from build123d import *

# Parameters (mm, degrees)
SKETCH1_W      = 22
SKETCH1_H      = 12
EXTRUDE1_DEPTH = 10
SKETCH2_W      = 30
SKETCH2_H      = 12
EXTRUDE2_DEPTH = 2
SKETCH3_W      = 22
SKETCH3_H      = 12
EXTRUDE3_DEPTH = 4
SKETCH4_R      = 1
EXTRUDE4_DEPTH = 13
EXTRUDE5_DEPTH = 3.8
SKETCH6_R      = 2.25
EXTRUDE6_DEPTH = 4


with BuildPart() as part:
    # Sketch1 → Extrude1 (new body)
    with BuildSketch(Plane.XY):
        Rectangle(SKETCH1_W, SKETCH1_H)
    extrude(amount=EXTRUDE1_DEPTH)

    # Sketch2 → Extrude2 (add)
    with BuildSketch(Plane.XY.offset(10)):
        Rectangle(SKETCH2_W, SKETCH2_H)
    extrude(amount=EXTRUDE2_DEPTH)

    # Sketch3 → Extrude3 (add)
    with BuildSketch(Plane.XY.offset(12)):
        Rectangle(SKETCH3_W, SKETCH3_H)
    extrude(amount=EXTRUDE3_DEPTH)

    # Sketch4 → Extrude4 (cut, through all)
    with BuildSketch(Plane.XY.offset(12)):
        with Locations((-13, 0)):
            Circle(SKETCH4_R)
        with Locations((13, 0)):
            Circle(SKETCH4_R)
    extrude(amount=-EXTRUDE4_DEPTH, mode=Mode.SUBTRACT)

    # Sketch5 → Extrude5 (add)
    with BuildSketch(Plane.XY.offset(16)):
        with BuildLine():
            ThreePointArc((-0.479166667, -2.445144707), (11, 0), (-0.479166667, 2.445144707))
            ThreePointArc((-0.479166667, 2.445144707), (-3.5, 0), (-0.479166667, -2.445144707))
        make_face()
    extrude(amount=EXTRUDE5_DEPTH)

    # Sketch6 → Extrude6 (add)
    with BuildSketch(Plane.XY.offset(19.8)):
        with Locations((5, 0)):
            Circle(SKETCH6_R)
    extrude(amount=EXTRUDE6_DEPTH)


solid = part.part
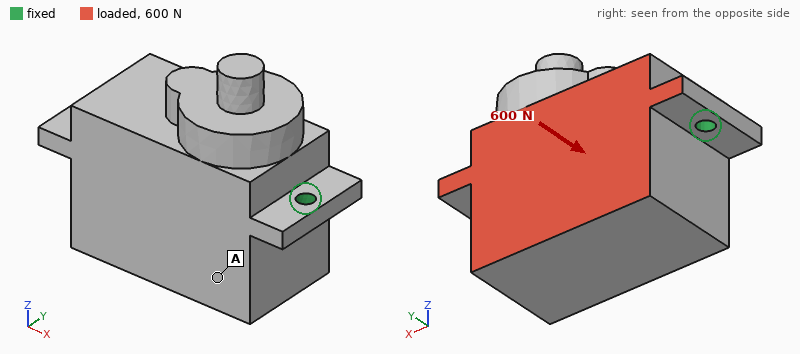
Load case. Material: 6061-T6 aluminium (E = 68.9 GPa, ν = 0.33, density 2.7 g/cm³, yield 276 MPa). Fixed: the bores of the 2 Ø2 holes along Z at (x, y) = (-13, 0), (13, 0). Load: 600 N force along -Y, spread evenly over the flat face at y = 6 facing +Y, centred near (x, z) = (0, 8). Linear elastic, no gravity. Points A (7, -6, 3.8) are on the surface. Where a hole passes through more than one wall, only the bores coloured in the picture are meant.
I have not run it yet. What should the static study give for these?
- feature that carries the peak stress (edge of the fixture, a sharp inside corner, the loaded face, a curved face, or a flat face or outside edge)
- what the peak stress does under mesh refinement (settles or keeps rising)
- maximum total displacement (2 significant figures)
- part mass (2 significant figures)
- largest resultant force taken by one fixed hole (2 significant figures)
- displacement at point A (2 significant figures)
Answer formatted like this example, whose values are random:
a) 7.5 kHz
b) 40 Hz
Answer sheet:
a) edge of the fixture
b) keeps rising
c) 36 µm
d) 13 g
e) 300 N
f) 27 µm
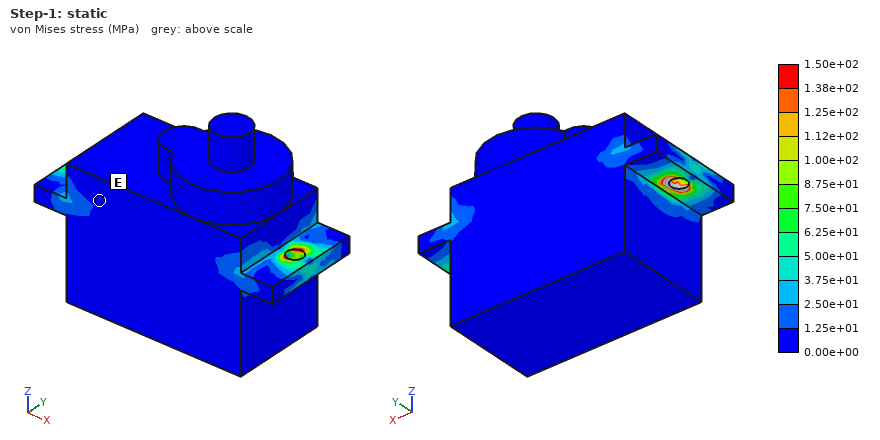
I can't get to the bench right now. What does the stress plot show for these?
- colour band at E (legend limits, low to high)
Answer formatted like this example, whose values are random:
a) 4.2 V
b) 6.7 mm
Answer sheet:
a) 0.00e+00 to 1.25e+01 MPa
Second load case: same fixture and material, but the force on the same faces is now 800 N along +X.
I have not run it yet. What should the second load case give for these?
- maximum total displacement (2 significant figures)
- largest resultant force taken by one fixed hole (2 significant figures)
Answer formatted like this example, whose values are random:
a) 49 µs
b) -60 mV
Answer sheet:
a) 5.0 µm
b) 450 N
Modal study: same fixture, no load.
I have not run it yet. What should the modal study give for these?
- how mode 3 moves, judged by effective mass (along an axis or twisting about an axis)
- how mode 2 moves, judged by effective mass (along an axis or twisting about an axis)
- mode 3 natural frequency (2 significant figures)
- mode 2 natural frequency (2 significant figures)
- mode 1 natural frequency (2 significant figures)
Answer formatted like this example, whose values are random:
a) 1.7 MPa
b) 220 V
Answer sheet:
a) along Y
b) along Z
c) 20 kHz
d) 18 kHz
e) 5400 Hz
